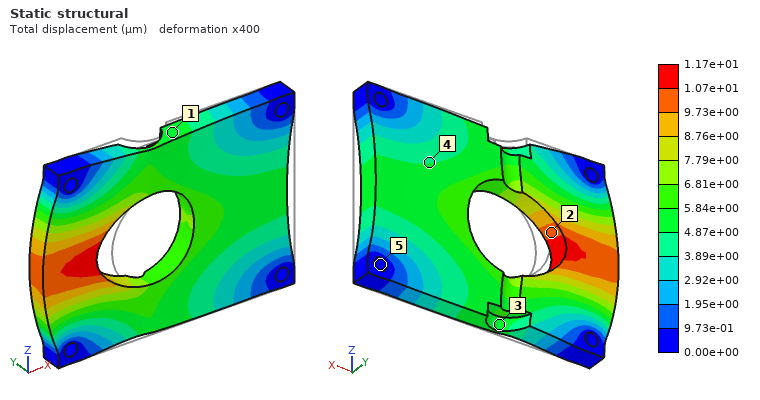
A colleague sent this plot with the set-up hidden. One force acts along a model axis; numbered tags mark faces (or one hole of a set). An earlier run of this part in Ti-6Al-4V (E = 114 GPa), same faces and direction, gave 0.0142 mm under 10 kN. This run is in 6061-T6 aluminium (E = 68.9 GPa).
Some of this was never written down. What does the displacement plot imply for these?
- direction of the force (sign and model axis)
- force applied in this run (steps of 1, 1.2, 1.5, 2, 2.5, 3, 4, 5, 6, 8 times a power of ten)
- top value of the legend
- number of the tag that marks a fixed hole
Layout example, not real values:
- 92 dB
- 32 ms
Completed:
- -X
- 5 kN
- 1.17e+01 µm
- 5
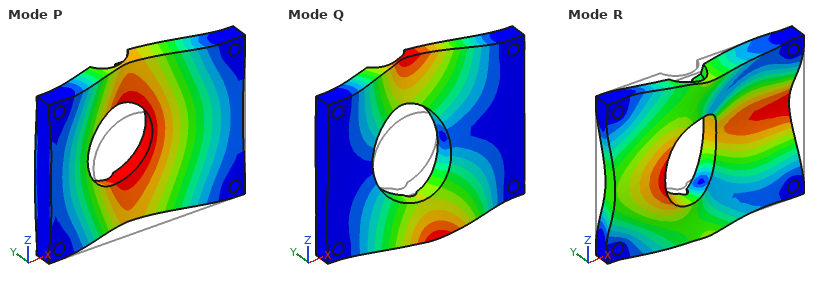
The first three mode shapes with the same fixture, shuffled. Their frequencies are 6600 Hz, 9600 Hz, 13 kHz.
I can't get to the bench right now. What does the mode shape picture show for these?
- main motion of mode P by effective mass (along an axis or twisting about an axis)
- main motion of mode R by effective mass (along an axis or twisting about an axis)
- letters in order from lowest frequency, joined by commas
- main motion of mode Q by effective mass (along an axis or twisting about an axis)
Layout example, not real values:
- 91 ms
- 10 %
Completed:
- along Y
- twisting about Z
- P, Q, R
- twisting about X
